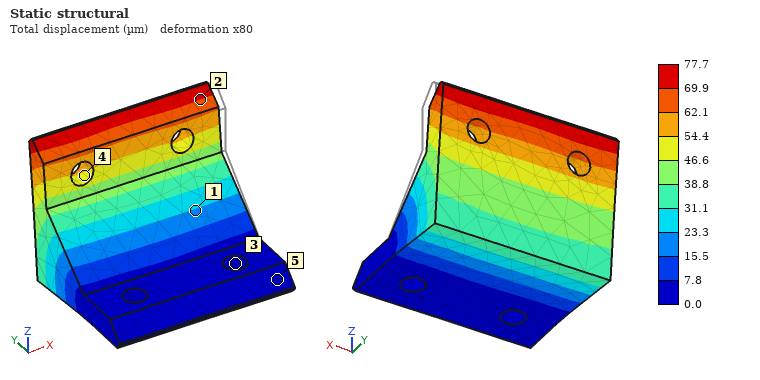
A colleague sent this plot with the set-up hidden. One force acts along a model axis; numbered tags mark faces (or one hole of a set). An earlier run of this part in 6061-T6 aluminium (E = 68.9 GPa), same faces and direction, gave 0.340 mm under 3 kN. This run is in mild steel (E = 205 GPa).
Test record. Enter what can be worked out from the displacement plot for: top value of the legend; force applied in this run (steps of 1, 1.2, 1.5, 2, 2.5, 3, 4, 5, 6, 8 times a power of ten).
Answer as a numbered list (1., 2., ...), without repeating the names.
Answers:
1. 77.7 µm
2. 2 kN
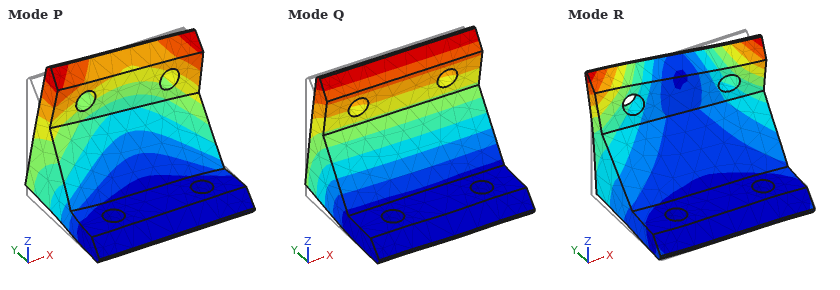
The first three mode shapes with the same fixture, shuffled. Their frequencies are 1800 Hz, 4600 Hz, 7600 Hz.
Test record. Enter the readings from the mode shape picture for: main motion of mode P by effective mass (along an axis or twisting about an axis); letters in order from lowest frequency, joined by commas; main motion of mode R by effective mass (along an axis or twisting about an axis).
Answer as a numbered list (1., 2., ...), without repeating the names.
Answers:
1. along X
2. Q, P, R
3. along X
